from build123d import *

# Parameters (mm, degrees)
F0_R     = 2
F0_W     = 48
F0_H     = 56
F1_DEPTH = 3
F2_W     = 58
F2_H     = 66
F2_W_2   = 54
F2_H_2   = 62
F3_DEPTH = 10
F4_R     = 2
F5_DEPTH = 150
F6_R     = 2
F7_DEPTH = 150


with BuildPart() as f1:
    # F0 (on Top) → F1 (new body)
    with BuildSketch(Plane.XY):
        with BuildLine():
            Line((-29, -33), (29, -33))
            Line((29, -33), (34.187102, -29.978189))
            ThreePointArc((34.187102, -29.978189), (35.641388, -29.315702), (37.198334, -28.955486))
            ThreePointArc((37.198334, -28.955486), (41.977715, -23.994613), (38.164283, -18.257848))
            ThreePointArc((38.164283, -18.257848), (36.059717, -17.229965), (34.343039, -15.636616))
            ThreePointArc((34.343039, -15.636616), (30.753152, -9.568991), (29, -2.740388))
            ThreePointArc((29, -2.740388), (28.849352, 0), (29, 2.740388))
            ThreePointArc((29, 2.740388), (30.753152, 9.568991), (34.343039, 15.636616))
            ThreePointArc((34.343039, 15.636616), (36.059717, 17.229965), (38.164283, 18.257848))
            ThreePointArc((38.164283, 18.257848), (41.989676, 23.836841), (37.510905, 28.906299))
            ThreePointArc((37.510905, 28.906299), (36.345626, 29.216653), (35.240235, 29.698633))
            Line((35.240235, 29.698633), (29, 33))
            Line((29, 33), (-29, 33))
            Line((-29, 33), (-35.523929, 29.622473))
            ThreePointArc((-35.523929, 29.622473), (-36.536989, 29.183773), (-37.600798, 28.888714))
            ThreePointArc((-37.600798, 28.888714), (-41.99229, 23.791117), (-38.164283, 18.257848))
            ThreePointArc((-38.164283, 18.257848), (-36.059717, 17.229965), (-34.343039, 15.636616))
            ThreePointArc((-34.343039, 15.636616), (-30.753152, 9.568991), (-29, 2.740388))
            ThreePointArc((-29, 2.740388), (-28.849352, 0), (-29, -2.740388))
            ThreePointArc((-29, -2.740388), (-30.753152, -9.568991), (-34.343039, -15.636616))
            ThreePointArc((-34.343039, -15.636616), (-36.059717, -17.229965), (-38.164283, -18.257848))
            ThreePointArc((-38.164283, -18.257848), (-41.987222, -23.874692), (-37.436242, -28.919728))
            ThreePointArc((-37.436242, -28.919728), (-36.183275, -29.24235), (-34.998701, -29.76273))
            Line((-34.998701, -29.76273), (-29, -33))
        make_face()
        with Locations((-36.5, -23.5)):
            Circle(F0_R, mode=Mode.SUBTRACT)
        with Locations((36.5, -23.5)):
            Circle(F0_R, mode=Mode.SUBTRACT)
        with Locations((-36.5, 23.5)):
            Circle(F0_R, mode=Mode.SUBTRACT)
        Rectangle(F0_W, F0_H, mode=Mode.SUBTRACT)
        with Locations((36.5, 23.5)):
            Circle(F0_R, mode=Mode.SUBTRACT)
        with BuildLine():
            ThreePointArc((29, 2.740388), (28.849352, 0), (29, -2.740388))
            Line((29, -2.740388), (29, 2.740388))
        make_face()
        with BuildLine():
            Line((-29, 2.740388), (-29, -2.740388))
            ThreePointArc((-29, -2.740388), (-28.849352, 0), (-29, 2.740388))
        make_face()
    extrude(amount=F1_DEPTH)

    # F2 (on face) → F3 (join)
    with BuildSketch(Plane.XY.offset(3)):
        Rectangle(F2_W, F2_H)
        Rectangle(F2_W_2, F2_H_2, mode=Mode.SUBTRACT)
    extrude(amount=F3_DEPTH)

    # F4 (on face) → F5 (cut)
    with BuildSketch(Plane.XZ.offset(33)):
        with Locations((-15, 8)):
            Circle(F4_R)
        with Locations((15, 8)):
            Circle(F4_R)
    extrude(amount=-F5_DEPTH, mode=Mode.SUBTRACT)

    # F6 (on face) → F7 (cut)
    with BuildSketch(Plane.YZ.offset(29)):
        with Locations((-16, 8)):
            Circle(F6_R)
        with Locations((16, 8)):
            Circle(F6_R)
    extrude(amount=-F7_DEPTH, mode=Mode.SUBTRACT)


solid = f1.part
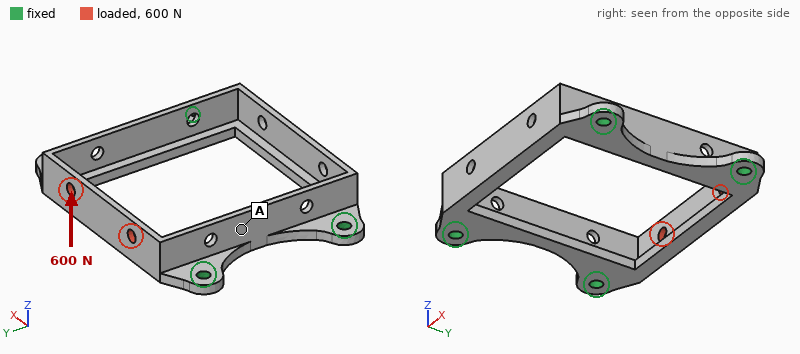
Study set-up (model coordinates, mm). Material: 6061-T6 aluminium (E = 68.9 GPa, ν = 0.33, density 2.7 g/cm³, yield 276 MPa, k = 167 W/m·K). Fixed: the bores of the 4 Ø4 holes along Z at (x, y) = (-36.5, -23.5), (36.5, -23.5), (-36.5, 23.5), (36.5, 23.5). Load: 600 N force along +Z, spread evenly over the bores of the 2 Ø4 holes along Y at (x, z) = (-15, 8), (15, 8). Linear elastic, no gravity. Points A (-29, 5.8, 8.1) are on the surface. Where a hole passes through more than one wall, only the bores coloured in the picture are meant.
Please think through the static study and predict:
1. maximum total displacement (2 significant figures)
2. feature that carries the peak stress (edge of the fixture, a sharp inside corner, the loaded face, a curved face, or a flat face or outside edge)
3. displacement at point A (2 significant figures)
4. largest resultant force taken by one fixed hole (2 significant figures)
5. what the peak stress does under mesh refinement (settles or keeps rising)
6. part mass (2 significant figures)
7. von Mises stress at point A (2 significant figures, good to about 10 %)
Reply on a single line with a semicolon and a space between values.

88 µm; edge of the fixture; 15 µm; 440 N; keeps rising; 27 g; 10 MPa
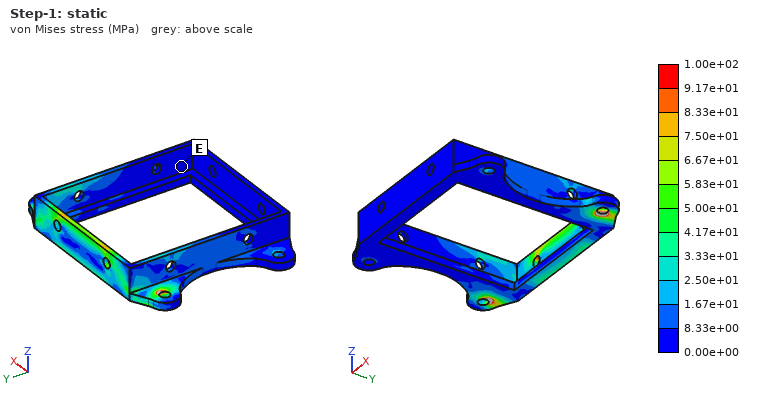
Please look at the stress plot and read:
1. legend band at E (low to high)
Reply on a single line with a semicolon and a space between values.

0.00e+00 to 8.33e+00 MPa
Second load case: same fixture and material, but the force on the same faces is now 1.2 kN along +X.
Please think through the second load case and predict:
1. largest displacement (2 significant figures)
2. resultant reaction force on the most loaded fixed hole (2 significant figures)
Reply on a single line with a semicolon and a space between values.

23 µm; 660 N
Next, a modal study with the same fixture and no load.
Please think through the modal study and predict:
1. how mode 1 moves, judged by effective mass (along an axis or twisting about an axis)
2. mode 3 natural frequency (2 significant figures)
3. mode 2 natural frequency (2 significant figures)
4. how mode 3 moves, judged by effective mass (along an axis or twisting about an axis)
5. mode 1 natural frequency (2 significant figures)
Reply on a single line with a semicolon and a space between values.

along Y; 6400 Hz; 5200 Hz; along Z; 5000 Hz
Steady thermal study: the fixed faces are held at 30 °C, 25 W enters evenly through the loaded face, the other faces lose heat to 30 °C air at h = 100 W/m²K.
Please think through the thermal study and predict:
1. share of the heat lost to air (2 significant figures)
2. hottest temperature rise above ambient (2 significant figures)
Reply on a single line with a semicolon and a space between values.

33 %; 43 K
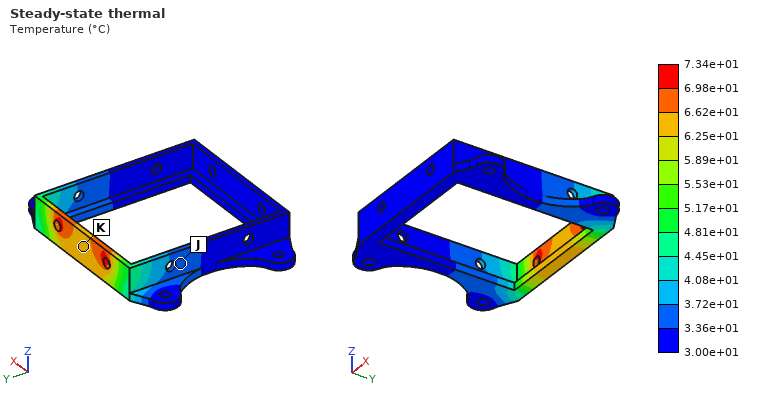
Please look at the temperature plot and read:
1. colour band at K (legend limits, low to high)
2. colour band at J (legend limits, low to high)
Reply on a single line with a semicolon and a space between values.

6.25e+01 to 6.62e+01 °C; 3.36e+01 to 3.72e+01 °C
